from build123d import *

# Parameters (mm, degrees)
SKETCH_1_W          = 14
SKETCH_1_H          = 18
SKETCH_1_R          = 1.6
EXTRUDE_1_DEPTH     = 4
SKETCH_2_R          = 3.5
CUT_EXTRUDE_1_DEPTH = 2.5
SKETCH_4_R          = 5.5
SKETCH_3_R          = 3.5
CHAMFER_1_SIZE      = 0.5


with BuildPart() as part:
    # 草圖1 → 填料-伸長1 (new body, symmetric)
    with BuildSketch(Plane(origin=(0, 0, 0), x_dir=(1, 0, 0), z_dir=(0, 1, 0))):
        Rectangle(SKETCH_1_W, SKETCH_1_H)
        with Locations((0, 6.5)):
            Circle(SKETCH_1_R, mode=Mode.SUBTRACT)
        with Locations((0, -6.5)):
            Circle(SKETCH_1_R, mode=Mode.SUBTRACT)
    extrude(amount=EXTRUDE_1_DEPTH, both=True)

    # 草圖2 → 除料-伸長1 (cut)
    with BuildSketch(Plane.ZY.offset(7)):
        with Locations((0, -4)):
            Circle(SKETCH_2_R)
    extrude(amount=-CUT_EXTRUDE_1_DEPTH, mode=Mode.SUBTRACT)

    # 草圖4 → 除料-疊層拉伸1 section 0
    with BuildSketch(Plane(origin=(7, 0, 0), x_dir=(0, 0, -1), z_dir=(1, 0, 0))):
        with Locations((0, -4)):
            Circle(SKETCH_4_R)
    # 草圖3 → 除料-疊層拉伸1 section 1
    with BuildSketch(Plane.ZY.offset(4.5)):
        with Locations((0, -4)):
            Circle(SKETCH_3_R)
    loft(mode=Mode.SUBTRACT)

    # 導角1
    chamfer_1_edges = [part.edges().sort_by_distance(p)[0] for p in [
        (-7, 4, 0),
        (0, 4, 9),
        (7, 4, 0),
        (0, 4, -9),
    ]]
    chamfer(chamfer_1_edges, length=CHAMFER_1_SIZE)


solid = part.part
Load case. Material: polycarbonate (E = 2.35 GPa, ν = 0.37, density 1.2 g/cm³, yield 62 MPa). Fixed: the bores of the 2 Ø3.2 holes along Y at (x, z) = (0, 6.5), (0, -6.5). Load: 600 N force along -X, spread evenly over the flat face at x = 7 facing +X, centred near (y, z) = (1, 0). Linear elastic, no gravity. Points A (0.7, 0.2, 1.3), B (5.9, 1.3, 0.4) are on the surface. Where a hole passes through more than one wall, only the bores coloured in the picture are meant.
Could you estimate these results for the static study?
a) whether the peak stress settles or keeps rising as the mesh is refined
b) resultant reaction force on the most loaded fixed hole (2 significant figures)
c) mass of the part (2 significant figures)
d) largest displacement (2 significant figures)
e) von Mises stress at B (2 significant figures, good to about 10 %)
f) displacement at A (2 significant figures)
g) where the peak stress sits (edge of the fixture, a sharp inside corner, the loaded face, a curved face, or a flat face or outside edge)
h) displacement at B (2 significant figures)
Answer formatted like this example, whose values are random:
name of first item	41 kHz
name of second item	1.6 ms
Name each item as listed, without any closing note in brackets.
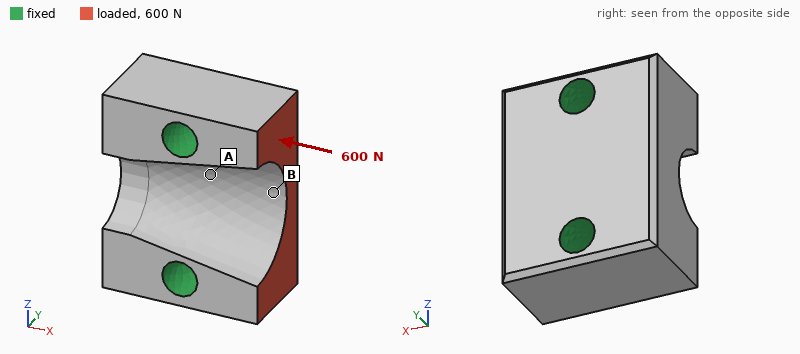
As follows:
whether the peak stress settles or keeps rising as the mesh is refined	keeps rising
resultant reaction force on the most loaded fixed hole	300 N
mass of the part	1.8 g
largest displacement	20 µm
von Mises stress at B	5.5 MPa
displacement at A	6.4 µm
where the peak stress sits	edge of the fixture
displacement at B	15 µm
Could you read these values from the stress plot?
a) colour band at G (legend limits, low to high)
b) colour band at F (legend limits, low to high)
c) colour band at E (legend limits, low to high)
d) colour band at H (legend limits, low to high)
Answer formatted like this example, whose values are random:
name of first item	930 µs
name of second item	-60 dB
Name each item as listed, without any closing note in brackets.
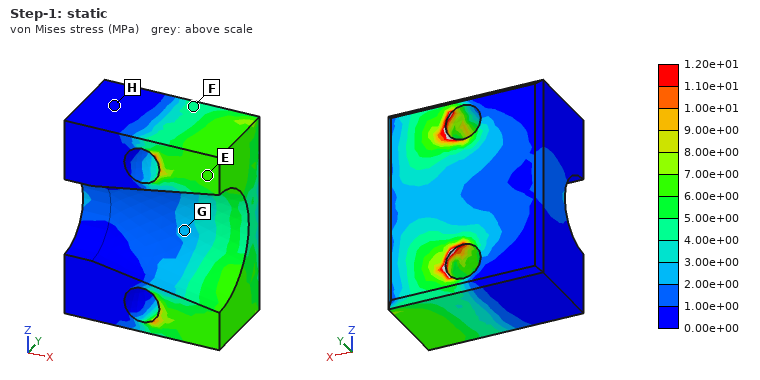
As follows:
colour band at G	2.00e+00 to 3.00e+00 MPa
colour band at F	4.00e+00 to 5.00e+00 MPa
colour band at E	6.00e+00 to 7.00e+00 MPa
colour band at H	0.00e+00 to 1.00e+00 MPa
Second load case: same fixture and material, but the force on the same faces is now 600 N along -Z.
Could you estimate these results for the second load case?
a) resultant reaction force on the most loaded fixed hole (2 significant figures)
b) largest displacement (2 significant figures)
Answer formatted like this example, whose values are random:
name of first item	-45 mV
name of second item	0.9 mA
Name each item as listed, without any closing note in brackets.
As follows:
resultant reaction force on the most loaded fixed hole	360 N
largest displacement	0.12 mm
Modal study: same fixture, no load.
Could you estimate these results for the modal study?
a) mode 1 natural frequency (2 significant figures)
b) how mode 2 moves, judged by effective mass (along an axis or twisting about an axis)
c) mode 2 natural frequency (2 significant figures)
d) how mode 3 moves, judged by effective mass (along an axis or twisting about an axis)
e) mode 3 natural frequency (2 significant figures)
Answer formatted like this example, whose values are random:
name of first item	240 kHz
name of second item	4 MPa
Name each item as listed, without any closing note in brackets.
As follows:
mode 1 natural frequency	22 kHz
how mode 2 moves, judged by effective mass	along Y
mode 2 natural frequency	24 kHz
how mode 3 moves, judged by effective mass	along Z
mode 3 natural frequency	26 kHz
